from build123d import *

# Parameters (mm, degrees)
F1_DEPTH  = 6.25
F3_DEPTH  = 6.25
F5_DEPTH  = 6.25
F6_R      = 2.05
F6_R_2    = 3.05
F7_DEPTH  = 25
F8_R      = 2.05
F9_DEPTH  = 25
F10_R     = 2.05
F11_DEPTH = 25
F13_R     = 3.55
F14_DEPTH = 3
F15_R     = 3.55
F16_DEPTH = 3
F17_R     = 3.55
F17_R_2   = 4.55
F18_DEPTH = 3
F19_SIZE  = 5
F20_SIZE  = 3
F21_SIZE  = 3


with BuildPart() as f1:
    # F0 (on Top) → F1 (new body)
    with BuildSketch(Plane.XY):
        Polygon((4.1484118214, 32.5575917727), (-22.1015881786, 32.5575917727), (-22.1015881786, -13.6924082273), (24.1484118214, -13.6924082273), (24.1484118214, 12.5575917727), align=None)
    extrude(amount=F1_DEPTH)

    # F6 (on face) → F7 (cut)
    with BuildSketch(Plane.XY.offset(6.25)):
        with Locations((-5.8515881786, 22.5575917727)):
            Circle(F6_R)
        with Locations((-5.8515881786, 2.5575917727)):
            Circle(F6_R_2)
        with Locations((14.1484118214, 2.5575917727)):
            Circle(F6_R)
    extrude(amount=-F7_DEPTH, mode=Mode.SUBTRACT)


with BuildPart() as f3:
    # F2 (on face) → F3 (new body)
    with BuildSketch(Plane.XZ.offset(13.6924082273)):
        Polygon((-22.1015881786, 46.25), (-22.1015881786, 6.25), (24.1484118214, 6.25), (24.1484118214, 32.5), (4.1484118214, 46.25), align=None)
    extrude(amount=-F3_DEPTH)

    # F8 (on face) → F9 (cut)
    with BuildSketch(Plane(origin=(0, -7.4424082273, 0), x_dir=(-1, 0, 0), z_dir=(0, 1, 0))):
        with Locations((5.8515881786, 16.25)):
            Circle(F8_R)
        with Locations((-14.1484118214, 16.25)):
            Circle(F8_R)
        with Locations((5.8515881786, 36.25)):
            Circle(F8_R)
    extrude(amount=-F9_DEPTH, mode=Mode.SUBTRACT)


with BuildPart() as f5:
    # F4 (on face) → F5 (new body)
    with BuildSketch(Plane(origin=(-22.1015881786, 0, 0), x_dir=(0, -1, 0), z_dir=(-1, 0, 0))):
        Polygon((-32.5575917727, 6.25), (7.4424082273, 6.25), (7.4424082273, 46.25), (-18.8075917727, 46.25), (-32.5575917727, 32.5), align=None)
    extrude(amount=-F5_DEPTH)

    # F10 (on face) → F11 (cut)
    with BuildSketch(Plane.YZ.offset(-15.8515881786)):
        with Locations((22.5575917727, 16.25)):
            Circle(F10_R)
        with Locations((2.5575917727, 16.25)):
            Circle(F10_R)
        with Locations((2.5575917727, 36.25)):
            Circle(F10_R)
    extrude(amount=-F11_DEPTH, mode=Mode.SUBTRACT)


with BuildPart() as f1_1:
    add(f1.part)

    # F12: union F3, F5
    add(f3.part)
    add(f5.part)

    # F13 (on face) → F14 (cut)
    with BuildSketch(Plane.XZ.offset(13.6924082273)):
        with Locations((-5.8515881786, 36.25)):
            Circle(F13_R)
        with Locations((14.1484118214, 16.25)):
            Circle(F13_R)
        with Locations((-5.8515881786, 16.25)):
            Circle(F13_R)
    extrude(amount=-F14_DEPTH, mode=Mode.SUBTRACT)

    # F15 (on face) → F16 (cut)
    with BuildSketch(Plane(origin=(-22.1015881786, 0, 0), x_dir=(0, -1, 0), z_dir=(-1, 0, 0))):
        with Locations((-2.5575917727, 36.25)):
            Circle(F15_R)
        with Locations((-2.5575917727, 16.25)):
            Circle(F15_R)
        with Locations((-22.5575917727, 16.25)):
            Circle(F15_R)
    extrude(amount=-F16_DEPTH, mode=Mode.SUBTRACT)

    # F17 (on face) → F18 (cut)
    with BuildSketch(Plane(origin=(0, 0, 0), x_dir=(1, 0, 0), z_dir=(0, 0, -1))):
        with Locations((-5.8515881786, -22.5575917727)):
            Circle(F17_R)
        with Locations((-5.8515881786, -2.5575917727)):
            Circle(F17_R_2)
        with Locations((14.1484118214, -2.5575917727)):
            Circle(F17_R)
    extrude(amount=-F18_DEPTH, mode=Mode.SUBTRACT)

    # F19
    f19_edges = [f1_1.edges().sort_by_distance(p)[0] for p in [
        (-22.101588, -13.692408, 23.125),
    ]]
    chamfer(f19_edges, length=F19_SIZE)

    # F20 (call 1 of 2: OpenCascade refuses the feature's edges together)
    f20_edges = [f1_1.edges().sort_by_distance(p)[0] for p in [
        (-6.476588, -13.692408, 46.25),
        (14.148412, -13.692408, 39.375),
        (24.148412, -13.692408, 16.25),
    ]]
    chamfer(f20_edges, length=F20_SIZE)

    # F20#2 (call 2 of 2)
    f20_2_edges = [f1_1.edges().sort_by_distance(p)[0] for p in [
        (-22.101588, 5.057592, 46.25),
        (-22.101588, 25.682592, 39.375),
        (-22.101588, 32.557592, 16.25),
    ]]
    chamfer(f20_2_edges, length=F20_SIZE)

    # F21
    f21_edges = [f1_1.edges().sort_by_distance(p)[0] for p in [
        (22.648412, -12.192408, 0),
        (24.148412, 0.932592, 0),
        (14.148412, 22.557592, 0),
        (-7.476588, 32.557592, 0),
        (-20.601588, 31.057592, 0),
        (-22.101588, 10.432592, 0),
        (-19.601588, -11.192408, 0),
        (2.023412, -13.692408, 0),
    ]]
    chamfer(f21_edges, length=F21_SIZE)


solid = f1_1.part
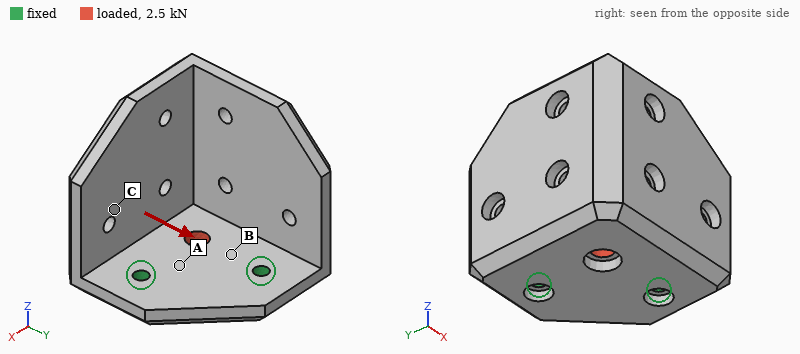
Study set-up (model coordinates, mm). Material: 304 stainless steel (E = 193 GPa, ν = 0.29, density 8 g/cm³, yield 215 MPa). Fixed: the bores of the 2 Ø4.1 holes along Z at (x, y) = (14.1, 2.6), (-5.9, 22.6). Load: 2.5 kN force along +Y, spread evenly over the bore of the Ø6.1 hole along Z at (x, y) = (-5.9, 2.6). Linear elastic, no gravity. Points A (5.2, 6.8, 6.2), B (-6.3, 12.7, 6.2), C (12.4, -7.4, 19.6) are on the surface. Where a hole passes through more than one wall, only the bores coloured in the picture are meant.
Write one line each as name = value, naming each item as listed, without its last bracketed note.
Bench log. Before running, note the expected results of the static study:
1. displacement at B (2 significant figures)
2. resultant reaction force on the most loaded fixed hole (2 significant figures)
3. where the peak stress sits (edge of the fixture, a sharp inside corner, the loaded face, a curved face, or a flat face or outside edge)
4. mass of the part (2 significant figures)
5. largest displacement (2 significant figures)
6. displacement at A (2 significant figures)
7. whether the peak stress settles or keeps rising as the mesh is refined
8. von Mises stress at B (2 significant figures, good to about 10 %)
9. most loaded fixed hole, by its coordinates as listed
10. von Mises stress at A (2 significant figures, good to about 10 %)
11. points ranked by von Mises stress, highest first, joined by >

displacement at B = 1.7 µm
resultant reaction force on the most loaded fixed hole = 2.0 kN
where the peak stress sits = edge of the fixture
mass of the part = 230 g
largest displacement = 5.8 µm
displacement at A = 1.1 µm
whether the peak stress settles or keeps rising as the mesh is refined = keeps rising
von Mises stress at B = 34 MPa
most loaded fixed hole, by its coordinates as listed = (-5.9, 22.6)
von Mises stress at A = 14 MPa
points ranked by von Mises stress, highest first, joined by > = B > A > C
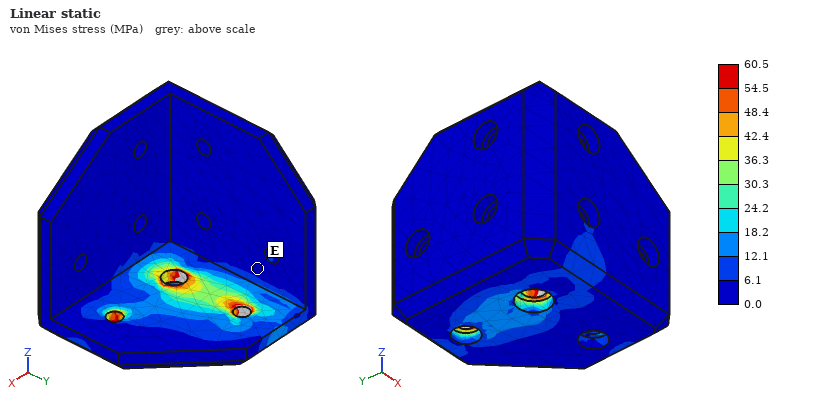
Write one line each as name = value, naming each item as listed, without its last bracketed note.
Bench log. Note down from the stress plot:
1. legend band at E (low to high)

legend band at E = 0.0 to 6.1 MPa
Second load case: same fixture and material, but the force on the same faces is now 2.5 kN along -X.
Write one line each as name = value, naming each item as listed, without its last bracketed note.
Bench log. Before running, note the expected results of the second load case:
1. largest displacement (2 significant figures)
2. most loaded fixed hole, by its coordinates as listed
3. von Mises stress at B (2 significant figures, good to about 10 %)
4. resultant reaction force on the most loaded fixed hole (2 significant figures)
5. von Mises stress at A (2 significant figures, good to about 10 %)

largest displacement = 5.8 µm
most loaded fixed hole, by its coordinates as listed = (14.1, 2.6)
von Mises stress at B = 11 MPa
resultant reaction force on the most loaded fixed hole = 2.0 kN
von Mises stress at A = 25 MPa
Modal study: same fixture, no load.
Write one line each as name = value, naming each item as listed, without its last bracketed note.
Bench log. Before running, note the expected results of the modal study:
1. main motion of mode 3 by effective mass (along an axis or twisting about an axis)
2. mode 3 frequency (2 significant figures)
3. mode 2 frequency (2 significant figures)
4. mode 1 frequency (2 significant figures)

main motion of mode 3 by effective mass = along Z
mode 3 frequency = 5600 Hz
mode 2 frequency = 2800 Hz
mode 1 frequency = 1300 Hz
